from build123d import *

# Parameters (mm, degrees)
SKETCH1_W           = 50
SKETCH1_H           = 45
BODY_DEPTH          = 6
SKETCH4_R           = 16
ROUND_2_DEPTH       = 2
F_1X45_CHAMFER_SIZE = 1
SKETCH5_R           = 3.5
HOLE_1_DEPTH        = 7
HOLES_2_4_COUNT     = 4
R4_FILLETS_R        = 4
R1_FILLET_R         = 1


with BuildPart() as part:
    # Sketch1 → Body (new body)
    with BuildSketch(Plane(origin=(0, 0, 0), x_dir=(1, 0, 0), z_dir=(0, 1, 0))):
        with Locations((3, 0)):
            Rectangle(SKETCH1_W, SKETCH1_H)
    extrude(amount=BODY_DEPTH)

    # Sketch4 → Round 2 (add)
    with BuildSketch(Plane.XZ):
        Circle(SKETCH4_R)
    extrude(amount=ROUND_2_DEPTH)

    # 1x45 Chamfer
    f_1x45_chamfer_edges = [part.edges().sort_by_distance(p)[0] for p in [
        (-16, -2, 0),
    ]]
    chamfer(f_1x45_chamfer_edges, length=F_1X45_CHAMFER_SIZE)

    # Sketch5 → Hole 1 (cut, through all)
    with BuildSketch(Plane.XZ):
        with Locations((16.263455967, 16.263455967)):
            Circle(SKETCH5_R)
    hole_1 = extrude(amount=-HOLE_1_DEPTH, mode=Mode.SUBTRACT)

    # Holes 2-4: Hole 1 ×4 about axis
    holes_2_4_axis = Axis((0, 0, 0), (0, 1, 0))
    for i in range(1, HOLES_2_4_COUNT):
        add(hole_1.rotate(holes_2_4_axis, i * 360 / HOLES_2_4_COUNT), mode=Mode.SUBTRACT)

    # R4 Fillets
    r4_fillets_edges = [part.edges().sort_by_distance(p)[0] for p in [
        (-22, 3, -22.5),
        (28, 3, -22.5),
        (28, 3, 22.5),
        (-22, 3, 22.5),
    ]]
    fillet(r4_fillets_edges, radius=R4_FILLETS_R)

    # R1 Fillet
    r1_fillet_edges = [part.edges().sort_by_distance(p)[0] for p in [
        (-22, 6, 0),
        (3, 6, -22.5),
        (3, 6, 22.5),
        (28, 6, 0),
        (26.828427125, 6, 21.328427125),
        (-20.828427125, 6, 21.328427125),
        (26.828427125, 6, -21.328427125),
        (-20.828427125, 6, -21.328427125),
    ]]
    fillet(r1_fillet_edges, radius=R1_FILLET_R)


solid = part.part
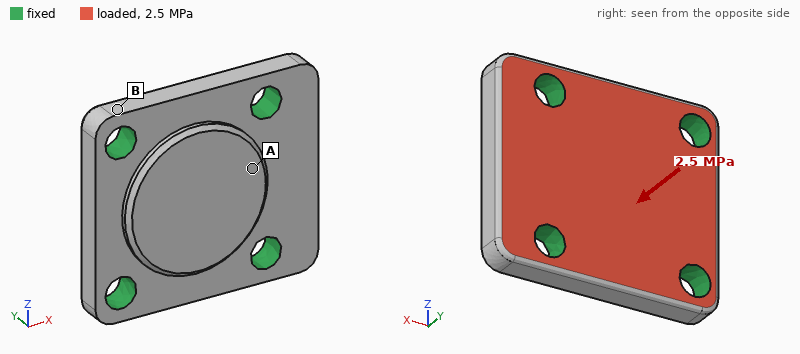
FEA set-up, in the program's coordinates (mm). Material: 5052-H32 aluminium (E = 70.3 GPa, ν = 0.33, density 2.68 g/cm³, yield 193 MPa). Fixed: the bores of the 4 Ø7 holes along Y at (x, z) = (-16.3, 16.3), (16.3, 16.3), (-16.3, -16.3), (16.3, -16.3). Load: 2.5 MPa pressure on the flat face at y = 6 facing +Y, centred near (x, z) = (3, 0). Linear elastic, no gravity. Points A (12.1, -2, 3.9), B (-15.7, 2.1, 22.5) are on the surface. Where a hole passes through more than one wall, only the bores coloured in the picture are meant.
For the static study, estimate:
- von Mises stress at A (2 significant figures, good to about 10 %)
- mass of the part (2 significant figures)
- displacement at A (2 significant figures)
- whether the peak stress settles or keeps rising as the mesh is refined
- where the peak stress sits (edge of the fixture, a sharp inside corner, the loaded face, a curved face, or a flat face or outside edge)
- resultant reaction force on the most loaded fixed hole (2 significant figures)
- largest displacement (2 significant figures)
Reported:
13 MPa
38 g
5.6 µm
keeps rising
edge of the fixture
1.4 kN
7.6 µm
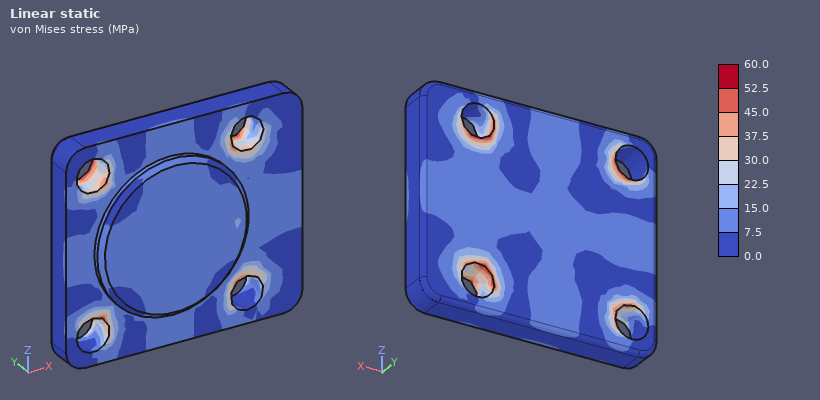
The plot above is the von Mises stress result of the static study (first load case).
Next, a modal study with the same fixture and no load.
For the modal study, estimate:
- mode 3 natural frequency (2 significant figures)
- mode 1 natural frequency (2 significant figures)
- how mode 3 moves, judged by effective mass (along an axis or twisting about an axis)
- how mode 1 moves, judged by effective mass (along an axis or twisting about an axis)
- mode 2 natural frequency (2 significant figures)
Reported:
34 kHz
24 kHz
twisting about X
along Y
27 kHz
